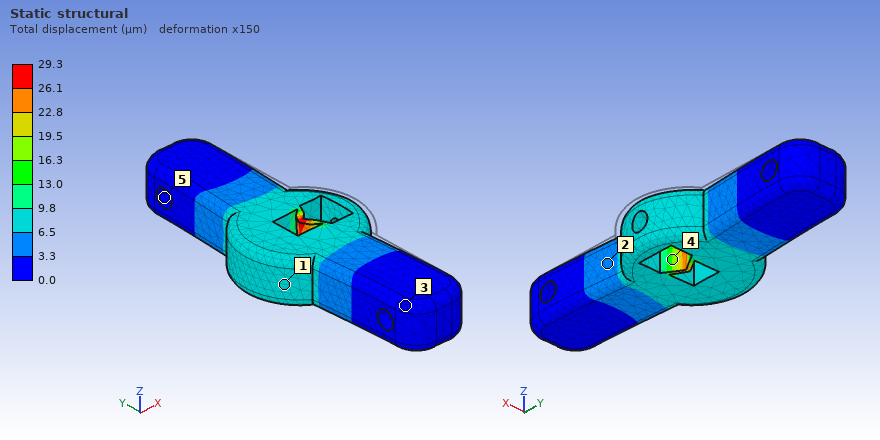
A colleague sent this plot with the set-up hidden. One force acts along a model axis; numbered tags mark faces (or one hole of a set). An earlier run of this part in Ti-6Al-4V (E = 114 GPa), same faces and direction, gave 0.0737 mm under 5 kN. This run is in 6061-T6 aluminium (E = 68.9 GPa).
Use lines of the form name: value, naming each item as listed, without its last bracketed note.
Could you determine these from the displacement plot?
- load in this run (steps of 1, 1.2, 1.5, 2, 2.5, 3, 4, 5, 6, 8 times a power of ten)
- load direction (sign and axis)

load in this run: 1.2 kN
load direction: -X
